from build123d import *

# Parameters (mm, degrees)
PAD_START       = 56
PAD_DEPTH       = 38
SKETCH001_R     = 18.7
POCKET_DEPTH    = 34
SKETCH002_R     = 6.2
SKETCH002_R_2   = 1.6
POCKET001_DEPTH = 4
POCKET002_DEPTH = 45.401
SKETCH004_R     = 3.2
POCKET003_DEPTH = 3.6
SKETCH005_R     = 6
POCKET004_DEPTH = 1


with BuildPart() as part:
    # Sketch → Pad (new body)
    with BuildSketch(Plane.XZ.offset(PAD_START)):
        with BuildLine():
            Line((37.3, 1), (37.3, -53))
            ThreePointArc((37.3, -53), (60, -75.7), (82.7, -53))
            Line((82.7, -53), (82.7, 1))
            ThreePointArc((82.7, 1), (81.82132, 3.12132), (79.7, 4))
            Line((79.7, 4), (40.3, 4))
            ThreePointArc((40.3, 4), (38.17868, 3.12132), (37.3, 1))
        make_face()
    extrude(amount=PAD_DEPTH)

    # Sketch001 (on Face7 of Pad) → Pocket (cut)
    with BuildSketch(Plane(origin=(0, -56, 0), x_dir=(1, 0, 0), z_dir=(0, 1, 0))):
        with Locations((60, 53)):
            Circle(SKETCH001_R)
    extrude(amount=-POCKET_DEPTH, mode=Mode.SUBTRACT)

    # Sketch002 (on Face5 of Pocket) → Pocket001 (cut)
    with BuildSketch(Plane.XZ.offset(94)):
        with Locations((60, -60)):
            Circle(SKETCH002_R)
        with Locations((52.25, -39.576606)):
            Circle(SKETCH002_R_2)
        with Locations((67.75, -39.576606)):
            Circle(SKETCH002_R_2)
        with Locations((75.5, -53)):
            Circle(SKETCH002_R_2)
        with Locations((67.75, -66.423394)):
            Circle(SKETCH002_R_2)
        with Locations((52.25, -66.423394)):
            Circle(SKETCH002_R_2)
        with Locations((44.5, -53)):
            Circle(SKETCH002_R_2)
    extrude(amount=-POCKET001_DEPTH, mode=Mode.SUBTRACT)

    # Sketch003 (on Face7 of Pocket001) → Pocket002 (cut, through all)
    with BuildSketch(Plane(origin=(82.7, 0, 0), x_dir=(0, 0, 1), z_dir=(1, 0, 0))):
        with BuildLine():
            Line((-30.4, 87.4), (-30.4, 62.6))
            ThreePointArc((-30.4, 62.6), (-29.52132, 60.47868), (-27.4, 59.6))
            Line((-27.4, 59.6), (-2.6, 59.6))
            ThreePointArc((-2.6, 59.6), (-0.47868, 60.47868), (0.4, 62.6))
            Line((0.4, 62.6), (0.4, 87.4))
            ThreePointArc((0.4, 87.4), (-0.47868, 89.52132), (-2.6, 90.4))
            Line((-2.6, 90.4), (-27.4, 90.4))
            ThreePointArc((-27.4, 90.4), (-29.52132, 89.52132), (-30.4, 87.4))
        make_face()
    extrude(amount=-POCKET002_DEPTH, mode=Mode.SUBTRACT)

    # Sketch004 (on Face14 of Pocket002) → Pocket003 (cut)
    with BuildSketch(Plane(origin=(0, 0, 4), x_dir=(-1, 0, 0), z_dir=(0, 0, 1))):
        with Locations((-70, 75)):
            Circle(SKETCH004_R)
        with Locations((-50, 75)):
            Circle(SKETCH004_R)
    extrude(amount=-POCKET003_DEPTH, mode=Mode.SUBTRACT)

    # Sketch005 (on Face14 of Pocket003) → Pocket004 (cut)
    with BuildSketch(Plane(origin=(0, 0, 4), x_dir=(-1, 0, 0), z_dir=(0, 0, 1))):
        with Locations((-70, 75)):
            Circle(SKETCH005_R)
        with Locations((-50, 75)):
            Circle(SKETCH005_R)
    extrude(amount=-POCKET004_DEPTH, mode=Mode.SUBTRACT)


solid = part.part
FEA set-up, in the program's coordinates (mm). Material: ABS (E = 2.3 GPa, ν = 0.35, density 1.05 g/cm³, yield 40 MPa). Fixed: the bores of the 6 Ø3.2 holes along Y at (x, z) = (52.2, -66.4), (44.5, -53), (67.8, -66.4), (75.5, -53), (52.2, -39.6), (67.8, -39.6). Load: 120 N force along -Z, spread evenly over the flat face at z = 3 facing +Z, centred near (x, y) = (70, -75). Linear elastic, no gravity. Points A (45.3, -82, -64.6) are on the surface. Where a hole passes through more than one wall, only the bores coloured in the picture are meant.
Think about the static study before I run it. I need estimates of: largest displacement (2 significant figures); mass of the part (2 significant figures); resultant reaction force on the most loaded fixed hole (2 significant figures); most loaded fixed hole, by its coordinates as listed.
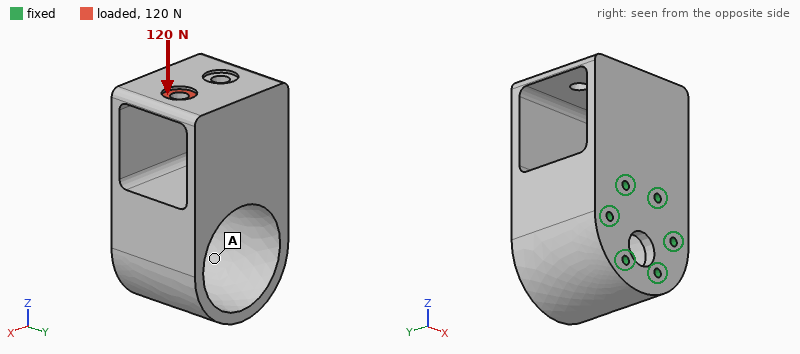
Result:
0.27 mm
50 g
61 N
(67.8, -39.6)
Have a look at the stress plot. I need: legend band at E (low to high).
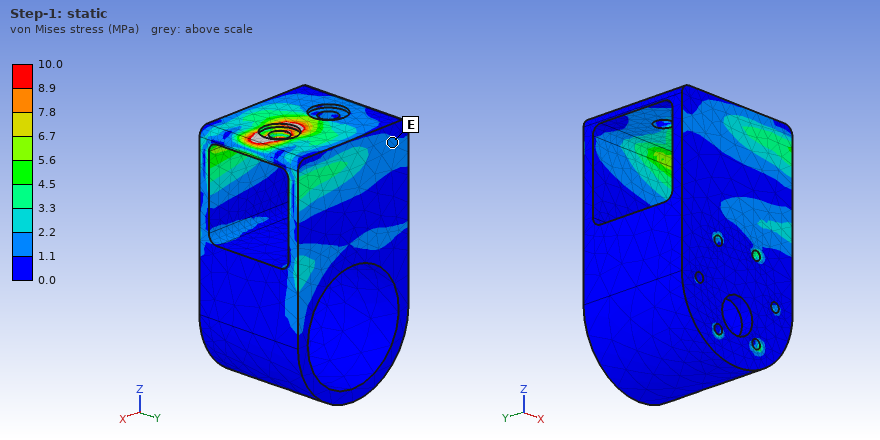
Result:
1.1 to 2.2 MPa
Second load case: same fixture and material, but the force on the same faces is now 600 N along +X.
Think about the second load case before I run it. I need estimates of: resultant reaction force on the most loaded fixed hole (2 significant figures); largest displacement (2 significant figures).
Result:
540 N
0.62 mm
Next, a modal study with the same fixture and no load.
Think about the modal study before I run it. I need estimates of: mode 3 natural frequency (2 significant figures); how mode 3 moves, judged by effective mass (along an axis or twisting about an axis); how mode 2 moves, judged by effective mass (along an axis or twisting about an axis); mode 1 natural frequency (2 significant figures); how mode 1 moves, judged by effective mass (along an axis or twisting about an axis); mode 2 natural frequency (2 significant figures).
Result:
1700 Hz
along Z
along X
660 Hz
along Y
1400 Hz
